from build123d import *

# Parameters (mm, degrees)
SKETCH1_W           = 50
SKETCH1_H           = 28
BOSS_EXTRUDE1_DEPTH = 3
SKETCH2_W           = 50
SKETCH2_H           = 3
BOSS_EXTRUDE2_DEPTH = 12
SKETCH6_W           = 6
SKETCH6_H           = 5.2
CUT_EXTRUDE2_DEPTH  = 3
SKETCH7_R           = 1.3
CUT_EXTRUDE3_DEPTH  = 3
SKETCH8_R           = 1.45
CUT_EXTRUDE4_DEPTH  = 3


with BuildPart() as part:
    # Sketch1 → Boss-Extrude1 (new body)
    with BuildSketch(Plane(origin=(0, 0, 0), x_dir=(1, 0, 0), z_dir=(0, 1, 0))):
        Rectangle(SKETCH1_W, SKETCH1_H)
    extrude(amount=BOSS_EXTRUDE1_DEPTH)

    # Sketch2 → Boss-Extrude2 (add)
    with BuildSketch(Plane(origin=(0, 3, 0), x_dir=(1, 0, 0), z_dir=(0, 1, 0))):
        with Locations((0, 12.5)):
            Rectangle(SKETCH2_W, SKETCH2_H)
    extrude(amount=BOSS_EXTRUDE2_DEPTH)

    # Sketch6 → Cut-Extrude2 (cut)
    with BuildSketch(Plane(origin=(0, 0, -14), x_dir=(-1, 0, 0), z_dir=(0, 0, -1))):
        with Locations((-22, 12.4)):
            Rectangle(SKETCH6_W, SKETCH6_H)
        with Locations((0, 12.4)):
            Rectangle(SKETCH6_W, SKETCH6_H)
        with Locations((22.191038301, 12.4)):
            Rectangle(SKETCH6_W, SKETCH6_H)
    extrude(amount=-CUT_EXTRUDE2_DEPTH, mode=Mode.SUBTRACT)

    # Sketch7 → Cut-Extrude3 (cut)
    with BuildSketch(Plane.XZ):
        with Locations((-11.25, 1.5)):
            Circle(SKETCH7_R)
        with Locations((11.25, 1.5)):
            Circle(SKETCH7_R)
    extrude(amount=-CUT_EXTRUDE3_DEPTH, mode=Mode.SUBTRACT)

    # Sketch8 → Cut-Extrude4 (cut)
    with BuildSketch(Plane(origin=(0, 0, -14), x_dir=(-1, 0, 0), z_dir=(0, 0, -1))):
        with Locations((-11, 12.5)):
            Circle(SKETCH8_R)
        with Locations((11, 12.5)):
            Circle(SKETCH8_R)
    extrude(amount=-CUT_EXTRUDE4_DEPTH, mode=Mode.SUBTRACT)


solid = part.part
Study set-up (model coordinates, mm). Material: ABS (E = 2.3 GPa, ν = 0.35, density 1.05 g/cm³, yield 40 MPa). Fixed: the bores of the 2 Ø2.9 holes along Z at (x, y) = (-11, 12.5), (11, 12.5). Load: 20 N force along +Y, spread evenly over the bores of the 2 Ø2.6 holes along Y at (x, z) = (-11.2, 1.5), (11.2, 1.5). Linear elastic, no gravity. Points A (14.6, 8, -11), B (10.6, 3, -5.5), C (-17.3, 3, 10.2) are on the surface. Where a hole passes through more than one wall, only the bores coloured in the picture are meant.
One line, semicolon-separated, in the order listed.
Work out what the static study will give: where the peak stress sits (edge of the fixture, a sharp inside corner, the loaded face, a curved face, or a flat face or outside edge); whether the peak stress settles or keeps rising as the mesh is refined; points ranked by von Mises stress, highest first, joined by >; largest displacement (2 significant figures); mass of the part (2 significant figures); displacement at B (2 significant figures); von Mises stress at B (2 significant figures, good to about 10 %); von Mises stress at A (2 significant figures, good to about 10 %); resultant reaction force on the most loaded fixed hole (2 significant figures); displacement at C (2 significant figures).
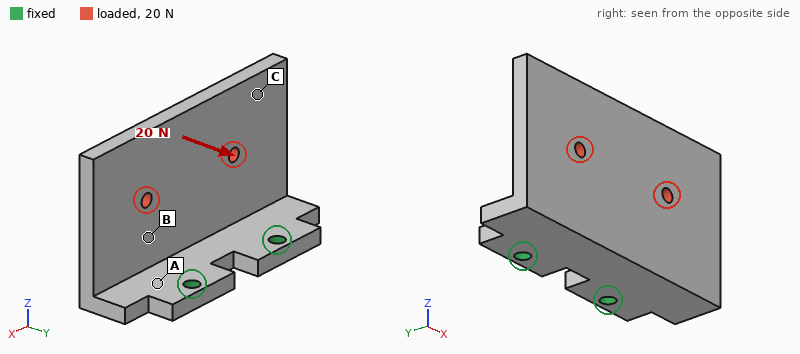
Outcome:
edge of the fixture; keeps rising; A > B > C; 0.57 mm; 5.9 g; 0.15 mm; 1.8 MPa; 4.9 MPa; 10 N; 0.47 mm
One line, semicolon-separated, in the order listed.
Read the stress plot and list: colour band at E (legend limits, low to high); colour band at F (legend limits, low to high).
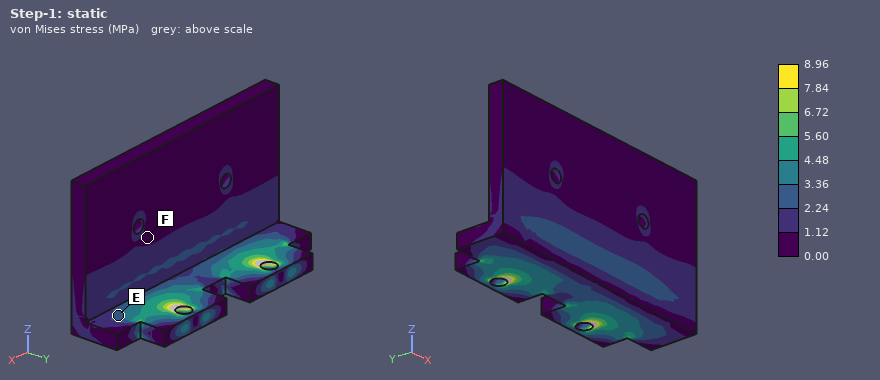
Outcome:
2.24 to 3.36 MPa; 0.00 to 1.12 MPa
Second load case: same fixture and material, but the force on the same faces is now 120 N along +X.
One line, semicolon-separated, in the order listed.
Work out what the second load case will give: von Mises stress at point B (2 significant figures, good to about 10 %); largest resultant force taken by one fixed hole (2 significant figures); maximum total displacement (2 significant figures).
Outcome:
5.8 MPa; 100 N; 0.70 mm
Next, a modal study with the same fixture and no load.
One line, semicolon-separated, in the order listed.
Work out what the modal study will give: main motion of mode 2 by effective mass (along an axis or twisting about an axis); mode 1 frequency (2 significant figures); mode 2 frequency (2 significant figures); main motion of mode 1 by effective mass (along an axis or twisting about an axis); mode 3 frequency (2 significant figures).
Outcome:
along X; 550 Hz; 990 Hz; along Y; 1600 Hz
